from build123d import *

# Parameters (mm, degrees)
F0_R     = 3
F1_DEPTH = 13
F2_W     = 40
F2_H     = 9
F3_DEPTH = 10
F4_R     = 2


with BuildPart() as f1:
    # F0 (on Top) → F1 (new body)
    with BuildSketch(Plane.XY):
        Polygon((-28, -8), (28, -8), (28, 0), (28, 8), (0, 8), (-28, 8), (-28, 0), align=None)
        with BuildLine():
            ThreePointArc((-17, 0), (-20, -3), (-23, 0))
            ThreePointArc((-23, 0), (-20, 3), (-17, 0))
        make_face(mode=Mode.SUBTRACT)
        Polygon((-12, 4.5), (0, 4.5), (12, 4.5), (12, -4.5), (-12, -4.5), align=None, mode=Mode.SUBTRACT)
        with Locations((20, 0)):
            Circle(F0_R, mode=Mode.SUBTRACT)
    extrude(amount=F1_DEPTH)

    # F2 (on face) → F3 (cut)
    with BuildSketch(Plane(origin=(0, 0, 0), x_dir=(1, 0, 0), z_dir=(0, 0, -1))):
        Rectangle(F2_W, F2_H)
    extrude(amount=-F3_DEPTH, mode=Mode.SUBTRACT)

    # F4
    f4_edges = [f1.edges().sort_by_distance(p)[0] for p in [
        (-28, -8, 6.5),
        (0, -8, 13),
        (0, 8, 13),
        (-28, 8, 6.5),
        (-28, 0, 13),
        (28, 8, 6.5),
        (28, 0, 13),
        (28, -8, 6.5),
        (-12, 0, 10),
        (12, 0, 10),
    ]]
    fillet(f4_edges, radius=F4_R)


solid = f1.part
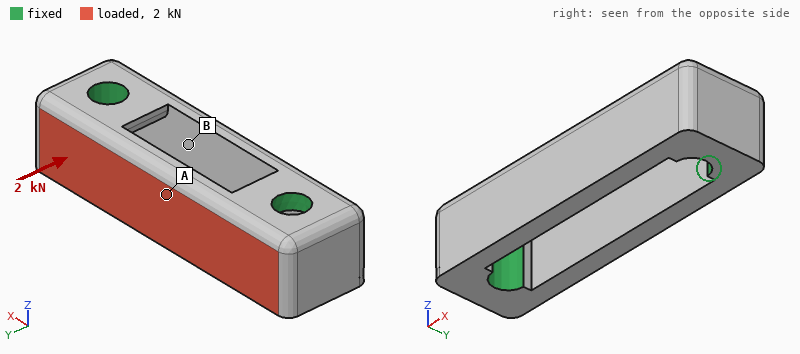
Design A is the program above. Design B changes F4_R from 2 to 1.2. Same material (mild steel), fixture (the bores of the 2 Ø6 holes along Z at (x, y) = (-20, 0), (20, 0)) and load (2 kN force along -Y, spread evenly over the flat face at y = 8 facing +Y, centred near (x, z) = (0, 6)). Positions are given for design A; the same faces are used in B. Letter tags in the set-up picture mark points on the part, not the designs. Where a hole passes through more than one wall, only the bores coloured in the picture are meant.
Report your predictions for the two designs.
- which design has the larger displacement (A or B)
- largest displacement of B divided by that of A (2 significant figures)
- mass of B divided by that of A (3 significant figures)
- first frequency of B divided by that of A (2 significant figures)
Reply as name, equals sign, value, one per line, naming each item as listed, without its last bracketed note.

which design has the larger displacement = A
largest displacement of B divided by that of A = 0.90
mass of B divided by that of A = 1.02
first frequency of B divided by that of A = 1.0
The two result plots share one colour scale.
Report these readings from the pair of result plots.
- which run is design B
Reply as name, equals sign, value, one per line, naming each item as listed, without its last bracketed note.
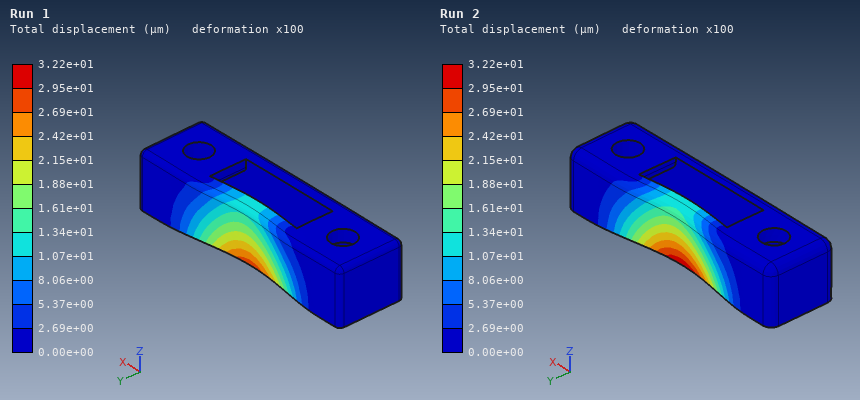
which run is design B = Run 1
